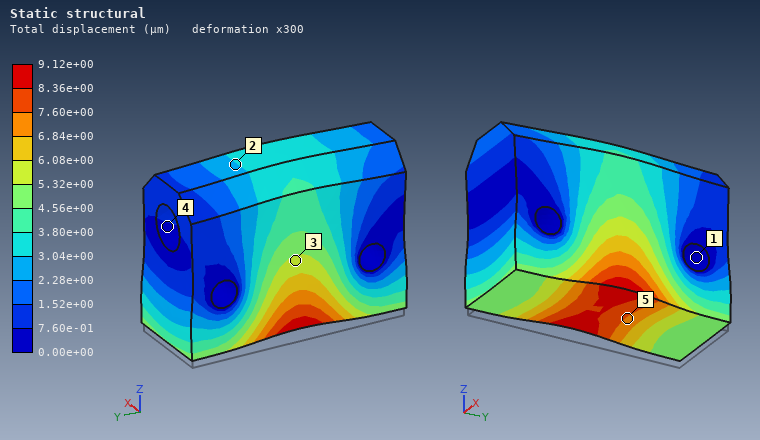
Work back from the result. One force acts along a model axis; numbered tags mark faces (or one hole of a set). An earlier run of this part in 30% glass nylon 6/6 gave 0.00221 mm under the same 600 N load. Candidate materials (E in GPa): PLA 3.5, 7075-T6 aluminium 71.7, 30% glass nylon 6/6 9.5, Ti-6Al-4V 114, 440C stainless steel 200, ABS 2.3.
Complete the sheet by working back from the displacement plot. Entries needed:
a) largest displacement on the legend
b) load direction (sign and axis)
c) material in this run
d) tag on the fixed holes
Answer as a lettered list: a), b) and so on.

a) 9.12e+00 µm
b) +Z
c) ABS
d) 1
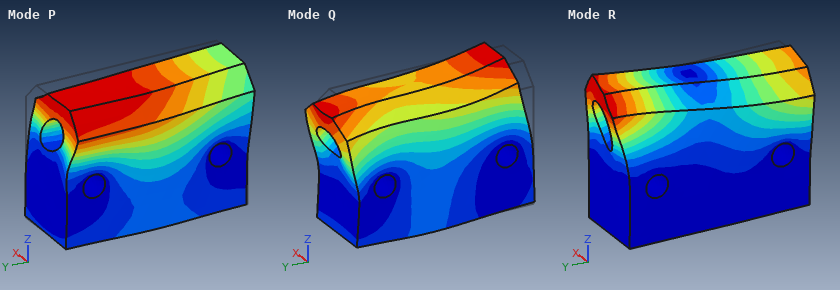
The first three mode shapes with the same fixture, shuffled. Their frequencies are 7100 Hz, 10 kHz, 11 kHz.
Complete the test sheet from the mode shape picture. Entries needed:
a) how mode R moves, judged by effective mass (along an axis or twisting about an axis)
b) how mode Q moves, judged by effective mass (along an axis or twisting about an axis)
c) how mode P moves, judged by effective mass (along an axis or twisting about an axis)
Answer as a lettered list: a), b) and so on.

a) twisting about Z
b) along Y
c) along X
